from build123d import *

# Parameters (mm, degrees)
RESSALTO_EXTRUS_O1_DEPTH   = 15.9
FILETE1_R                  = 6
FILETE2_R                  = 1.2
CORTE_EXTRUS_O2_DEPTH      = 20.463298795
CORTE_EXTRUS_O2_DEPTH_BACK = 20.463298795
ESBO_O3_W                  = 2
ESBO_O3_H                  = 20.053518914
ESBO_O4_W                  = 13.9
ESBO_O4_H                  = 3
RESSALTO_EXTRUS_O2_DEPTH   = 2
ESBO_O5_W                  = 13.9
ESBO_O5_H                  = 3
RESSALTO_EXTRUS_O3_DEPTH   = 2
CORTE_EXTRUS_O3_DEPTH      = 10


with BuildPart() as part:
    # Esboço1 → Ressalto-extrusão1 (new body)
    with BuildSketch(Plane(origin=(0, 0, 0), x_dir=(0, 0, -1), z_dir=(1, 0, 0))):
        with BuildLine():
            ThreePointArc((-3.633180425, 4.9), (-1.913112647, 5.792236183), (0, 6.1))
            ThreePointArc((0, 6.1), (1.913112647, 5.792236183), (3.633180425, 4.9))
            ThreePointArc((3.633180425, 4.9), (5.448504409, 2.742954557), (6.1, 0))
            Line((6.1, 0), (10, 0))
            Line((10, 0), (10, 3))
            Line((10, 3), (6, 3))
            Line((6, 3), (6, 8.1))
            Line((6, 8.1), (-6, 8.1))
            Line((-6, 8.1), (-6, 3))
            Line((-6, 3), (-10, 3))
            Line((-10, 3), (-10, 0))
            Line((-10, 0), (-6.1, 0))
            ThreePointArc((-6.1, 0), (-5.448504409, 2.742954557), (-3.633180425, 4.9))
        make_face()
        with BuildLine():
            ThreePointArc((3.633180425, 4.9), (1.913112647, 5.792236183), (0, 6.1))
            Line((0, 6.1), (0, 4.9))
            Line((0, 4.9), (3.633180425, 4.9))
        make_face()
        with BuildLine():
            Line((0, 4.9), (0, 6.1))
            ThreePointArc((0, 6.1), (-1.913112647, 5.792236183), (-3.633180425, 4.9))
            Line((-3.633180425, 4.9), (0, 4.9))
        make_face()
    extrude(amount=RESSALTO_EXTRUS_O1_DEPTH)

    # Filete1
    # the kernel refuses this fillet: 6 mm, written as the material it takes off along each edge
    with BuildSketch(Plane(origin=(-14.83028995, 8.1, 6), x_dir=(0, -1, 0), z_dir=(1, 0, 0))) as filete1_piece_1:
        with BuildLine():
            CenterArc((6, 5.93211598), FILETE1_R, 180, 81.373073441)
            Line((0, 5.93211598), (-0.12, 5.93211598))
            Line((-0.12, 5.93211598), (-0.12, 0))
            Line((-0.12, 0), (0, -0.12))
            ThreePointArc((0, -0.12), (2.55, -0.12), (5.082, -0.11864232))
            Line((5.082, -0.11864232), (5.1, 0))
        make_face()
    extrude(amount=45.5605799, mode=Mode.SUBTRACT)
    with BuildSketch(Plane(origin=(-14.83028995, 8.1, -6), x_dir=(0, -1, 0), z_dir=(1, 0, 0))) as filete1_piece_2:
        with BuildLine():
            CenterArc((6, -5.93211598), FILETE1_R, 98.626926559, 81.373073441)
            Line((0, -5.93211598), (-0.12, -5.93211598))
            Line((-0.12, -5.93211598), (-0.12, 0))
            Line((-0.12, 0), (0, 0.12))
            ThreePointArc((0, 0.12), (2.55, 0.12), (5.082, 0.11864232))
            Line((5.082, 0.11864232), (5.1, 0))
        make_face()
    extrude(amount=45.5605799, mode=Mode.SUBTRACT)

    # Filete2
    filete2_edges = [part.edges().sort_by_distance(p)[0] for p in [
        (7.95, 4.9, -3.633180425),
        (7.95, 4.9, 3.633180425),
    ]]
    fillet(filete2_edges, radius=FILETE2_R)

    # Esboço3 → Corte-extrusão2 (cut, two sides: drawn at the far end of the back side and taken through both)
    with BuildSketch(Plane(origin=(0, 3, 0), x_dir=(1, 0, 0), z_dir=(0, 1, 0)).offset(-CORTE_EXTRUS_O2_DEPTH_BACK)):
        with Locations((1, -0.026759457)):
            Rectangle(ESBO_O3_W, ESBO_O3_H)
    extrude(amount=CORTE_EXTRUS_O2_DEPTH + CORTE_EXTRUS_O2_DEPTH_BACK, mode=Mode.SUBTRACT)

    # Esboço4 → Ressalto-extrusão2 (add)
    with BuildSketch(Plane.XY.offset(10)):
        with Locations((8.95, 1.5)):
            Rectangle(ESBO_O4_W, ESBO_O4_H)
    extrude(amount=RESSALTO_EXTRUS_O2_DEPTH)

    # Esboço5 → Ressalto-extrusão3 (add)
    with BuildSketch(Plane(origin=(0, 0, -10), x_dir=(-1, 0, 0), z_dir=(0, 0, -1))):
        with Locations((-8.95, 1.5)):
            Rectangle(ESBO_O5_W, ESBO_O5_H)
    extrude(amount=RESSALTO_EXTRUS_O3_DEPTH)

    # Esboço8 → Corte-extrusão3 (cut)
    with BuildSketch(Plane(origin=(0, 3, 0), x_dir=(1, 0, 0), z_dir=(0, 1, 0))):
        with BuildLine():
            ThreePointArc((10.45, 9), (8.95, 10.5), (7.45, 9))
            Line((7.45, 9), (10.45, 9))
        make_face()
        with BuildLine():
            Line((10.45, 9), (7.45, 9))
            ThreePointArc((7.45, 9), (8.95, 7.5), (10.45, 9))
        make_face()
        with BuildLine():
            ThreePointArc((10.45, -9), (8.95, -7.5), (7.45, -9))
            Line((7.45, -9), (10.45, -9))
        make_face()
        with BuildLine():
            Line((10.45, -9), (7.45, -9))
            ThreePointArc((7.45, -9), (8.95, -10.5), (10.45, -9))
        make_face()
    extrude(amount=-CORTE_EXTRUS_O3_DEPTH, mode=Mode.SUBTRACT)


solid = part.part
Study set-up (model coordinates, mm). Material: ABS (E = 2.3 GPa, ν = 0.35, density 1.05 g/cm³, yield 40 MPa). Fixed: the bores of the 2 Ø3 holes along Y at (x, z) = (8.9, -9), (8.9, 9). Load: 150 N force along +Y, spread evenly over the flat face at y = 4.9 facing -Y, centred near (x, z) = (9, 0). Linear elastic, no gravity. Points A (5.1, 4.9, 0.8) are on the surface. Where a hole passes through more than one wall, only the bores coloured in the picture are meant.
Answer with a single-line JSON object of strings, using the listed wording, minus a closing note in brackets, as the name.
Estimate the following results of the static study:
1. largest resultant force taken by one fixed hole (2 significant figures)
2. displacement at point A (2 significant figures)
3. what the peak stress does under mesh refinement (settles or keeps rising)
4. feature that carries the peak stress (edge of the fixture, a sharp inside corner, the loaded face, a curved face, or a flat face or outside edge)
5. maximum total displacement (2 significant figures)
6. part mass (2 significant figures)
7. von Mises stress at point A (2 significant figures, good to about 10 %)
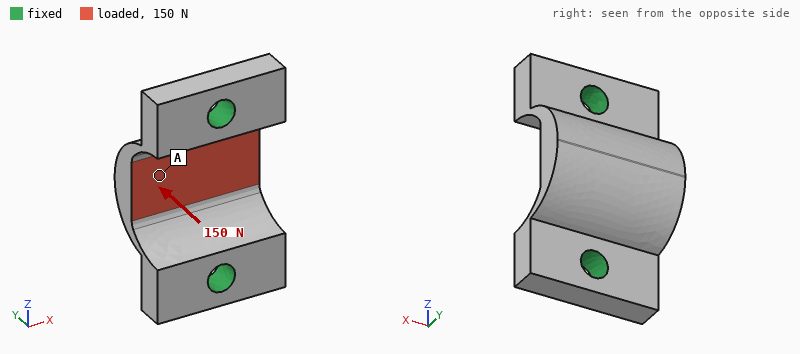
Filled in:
{"largest resultant force taken by one fixed hole": "93 N", "displacement at point A": "51 µm", "what the peak stress does under mesh refinement": "keeps rising", "feature that carries the peak stress": "edge of the fixture", "maximum total displacement": "59 µm", "part mass": "0.92 g", "von Mises stress at point A": "3.4 MPa"}
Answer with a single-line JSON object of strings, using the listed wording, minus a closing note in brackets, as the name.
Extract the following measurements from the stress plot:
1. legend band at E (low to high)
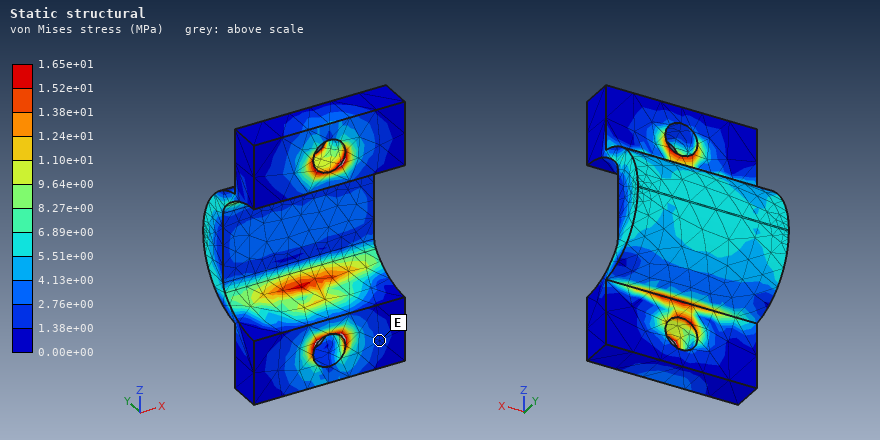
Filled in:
{"legend band at E": "1.38e+00 to 2.76e+00 MPa"}
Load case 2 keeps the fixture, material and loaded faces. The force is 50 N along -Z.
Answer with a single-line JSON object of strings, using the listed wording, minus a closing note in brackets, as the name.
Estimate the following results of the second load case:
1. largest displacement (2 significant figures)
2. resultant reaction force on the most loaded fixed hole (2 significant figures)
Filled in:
{"largest displacement": "33 µm", "resultant reaction force on the most loaded fixed hole": "26 N"}
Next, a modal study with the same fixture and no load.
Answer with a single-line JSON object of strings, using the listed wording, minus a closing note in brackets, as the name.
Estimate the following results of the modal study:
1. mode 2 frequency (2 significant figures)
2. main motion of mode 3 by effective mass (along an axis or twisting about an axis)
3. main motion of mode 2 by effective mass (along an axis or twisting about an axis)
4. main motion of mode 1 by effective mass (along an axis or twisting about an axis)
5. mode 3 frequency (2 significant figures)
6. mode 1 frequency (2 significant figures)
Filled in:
{"mode 2 frequency": "11 kHz", "main motion of mode 3 by effective mass": "along Y", "main motion of mode 2 by effective mass": "along Z", "main motion of mode 1 by effective mass": "along X", "mode 3 frequency": "14 kHz", "mode 1 frequency": "7300 Hz"}
